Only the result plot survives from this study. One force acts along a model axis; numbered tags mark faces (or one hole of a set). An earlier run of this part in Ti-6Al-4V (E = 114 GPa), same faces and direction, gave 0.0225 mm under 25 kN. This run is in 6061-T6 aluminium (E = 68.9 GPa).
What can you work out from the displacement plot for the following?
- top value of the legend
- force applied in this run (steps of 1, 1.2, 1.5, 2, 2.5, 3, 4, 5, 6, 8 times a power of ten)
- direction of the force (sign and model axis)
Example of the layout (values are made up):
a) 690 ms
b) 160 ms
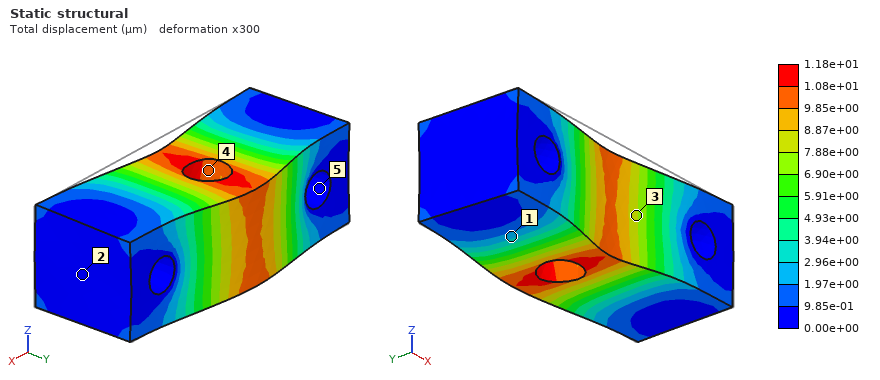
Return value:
a) 1.18e+01 µm
b) 8 kN
c) +Y
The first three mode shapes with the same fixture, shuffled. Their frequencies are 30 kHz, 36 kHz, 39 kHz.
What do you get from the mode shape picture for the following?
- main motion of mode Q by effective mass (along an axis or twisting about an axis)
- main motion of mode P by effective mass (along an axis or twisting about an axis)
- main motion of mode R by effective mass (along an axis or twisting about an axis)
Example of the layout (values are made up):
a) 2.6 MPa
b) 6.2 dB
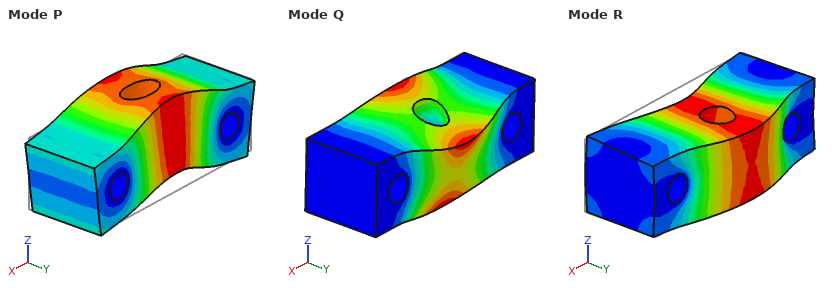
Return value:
a) twisting about X
b) along Z
c) along Y
